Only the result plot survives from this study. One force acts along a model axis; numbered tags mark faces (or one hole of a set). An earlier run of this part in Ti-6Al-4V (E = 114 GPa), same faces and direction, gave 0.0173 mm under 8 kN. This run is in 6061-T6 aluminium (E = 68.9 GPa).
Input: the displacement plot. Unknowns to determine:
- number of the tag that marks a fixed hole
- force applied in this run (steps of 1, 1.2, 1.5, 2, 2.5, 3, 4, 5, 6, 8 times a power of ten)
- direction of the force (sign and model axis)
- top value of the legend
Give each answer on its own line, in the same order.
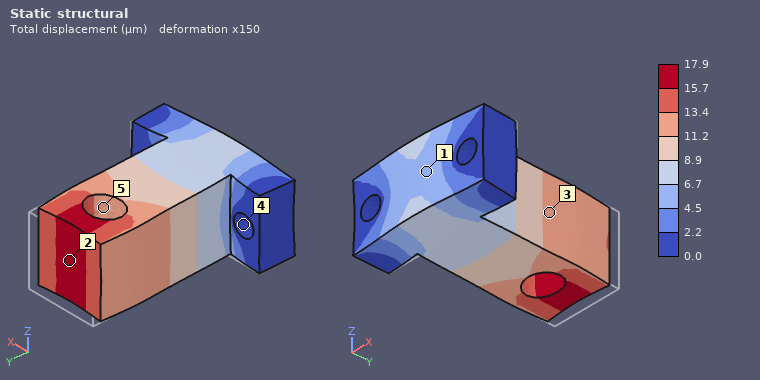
4
5 kN
-Y
17.9 µm
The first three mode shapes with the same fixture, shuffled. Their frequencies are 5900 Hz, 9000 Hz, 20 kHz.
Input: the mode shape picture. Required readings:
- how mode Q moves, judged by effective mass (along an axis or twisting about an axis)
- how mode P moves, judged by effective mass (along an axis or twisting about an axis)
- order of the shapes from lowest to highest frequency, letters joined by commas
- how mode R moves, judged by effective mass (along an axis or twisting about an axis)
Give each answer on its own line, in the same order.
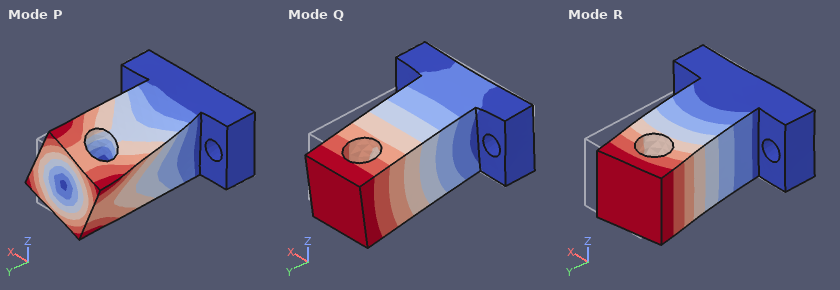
along Z
twisting about Y
Q, R, P
along X
